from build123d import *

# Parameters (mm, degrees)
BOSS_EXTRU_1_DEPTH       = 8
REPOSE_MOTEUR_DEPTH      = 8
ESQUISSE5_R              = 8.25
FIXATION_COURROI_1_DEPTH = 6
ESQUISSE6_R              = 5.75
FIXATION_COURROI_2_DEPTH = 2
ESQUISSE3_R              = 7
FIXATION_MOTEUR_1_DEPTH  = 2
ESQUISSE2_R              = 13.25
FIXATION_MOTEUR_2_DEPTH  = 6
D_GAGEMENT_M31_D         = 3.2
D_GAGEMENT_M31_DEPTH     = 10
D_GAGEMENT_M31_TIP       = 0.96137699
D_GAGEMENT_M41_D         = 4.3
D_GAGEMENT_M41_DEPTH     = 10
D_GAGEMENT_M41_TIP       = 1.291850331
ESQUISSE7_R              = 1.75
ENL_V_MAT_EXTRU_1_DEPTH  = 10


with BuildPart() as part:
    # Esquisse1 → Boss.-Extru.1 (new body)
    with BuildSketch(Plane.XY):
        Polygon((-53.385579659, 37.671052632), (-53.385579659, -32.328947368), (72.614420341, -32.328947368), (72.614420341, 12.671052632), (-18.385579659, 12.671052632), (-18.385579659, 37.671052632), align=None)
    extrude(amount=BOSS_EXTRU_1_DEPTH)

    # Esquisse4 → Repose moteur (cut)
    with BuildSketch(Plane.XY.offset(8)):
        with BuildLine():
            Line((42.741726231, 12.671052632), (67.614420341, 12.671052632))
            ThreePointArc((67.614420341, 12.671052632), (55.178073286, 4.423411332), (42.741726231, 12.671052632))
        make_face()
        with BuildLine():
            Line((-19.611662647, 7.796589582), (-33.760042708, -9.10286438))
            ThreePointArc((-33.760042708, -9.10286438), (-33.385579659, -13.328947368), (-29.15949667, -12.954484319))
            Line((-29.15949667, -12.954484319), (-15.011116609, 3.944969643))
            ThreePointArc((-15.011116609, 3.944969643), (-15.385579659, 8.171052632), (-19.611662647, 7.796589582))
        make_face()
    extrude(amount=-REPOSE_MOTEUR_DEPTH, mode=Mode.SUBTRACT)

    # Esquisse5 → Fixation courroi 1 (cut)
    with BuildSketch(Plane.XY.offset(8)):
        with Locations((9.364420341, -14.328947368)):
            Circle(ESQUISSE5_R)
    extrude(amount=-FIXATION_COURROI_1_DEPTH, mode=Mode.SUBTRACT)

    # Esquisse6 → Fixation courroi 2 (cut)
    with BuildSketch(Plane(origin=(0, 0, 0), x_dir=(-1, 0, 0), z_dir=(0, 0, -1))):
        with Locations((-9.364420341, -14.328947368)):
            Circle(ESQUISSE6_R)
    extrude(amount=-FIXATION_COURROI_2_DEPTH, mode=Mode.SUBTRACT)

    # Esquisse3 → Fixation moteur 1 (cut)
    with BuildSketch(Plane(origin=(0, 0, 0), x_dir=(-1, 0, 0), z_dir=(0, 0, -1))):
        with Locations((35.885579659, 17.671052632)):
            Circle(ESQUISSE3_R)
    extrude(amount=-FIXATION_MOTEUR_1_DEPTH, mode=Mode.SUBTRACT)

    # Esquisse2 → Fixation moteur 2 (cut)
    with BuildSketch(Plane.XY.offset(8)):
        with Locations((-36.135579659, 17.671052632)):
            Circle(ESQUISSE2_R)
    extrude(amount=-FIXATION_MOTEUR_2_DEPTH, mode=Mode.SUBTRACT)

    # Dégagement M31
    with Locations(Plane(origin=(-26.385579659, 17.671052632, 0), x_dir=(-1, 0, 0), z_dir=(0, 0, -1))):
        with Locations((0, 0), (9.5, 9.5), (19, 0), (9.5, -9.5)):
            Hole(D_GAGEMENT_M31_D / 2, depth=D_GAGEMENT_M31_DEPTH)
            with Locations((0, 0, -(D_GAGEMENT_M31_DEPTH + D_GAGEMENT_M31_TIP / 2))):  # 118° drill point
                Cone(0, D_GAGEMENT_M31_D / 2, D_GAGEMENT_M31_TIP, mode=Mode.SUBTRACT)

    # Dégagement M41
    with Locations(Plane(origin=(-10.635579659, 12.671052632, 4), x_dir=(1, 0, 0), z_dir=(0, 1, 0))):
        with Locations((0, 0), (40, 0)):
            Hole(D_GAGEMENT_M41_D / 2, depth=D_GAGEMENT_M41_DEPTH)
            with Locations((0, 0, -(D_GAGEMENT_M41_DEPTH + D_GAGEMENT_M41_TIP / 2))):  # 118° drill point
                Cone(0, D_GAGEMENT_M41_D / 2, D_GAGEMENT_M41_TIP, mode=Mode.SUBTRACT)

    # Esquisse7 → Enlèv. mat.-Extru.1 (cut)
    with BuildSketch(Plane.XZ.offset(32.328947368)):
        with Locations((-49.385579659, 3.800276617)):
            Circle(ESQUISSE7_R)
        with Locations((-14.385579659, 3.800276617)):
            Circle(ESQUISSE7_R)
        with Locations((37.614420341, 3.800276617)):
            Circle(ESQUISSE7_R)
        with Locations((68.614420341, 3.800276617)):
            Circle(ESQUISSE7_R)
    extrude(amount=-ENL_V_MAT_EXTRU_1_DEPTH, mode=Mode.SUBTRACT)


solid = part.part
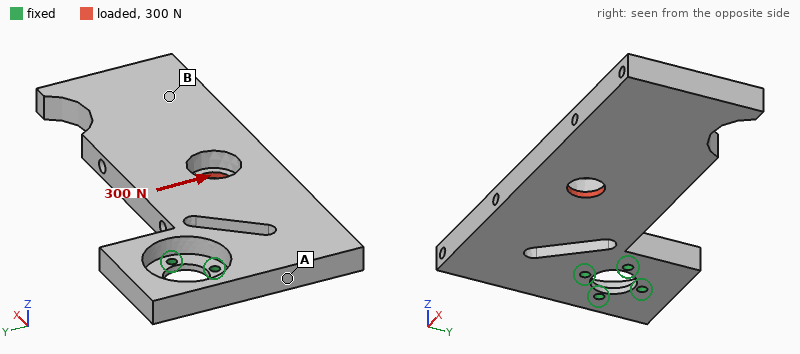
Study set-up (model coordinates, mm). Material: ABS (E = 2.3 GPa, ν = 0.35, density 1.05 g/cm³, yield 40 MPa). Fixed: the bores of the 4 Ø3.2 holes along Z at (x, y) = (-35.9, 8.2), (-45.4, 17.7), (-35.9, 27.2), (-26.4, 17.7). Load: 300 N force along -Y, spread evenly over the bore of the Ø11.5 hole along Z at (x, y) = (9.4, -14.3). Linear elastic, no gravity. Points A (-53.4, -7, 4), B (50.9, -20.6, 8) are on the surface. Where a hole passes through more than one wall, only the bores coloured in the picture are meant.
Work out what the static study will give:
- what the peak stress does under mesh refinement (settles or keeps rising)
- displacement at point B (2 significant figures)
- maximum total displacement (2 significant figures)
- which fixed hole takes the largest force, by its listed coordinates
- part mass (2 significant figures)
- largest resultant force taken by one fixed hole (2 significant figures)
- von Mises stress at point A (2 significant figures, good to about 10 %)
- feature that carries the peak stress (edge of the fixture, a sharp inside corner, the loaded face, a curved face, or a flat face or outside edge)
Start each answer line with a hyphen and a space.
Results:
- keeps rising
- 1.2 mm
- 1.7 mm
- (-26.4, 17.7)
- 46 g
- 500 N
- 6.2 MPa
- edge of the fixture
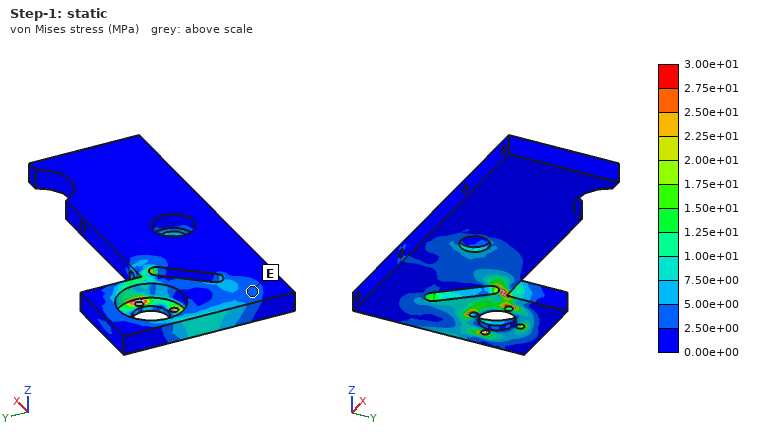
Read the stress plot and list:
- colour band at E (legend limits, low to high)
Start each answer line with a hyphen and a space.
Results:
- 2.50e+00 to 5.00e+00 MPa
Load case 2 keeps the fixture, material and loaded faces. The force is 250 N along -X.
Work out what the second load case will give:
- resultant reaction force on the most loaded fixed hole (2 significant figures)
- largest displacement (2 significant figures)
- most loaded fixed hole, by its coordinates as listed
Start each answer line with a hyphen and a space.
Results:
- 280 N
- 1.6 mm
- (-35.9, 8.2)
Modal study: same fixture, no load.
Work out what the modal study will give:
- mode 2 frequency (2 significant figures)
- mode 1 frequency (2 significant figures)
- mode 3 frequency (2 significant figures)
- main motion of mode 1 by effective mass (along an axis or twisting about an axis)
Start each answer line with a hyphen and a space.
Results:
- 370 Hz
- 97 Hz
- 390 Hz
- along Z
